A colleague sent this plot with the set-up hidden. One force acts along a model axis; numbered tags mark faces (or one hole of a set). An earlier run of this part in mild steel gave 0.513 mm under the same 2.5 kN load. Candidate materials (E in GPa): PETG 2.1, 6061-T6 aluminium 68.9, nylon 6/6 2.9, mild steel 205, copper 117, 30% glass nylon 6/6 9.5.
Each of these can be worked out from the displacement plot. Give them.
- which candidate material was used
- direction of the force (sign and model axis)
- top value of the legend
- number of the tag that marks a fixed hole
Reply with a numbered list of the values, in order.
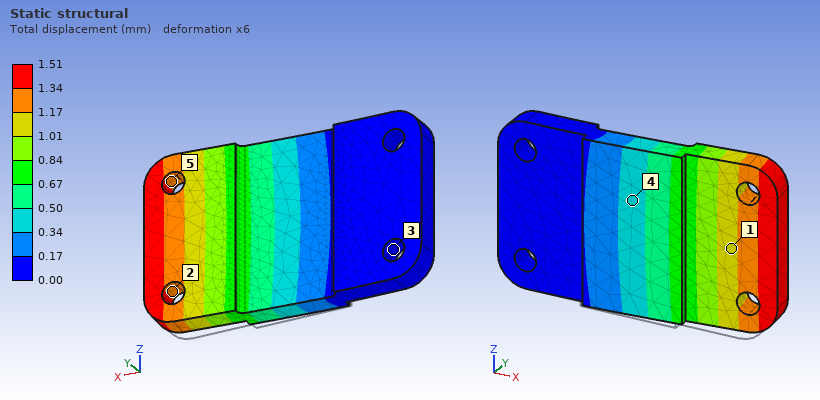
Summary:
1. 6061-T6 aluminium
2. +Y
3. 1.51 mm
4. 3
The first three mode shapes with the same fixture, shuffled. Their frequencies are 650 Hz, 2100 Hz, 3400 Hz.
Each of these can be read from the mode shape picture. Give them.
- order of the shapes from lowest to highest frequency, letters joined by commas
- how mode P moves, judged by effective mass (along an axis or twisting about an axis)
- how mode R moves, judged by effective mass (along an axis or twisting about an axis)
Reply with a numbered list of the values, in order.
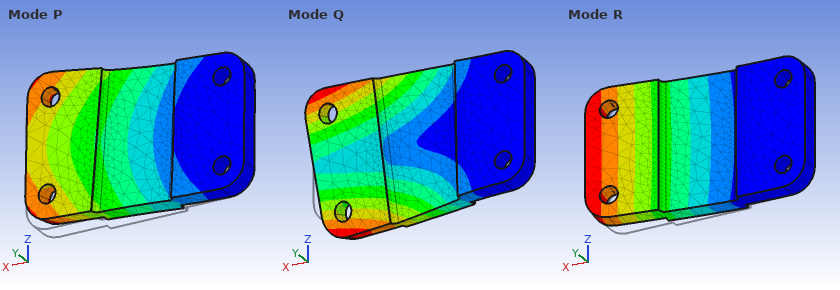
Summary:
1. R, Q, P
2. along Z
3. along Y
